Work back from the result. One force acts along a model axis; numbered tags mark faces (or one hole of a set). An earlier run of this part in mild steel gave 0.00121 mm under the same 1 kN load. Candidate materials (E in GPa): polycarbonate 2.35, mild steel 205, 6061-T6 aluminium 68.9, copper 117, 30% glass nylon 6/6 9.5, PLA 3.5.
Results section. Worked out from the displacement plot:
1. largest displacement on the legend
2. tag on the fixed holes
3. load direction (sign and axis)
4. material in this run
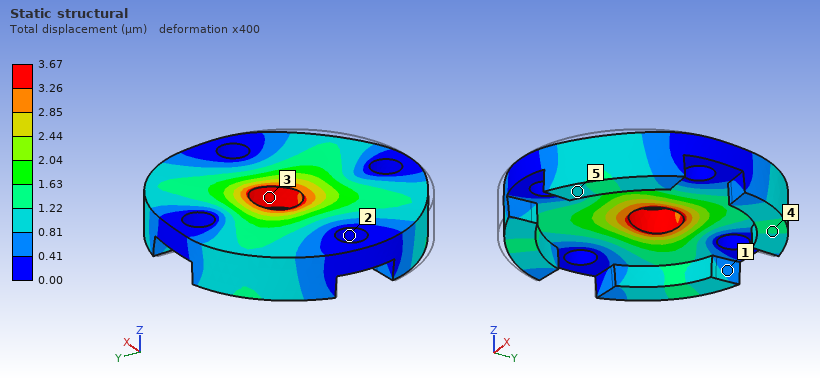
3.67 µm
2
+Y
6061-T6 aluminium
